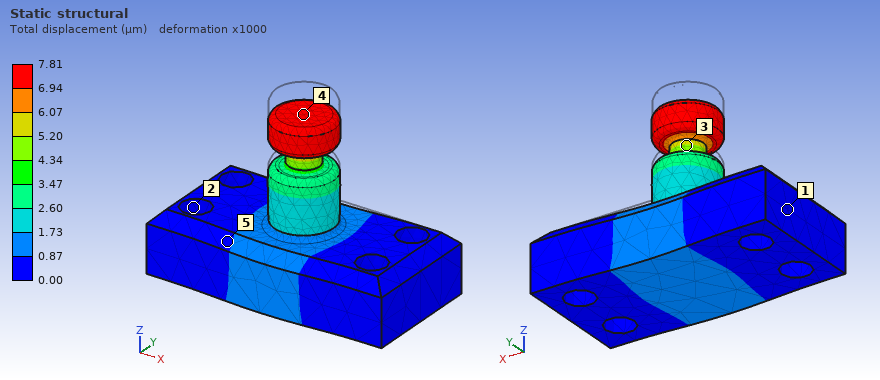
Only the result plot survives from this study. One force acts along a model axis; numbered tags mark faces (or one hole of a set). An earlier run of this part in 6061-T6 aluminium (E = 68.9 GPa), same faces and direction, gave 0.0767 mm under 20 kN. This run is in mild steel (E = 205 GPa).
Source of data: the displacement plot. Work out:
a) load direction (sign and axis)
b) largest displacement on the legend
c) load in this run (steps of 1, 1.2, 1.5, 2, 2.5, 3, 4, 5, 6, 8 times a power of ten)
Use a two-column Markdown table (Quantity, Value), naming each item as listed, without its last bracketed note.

| Quantity | Value |
|---|---|
| load direction | -Z |
| largest displacement on the legend | 7.81 µm |
| load in this run | 6 kN |
